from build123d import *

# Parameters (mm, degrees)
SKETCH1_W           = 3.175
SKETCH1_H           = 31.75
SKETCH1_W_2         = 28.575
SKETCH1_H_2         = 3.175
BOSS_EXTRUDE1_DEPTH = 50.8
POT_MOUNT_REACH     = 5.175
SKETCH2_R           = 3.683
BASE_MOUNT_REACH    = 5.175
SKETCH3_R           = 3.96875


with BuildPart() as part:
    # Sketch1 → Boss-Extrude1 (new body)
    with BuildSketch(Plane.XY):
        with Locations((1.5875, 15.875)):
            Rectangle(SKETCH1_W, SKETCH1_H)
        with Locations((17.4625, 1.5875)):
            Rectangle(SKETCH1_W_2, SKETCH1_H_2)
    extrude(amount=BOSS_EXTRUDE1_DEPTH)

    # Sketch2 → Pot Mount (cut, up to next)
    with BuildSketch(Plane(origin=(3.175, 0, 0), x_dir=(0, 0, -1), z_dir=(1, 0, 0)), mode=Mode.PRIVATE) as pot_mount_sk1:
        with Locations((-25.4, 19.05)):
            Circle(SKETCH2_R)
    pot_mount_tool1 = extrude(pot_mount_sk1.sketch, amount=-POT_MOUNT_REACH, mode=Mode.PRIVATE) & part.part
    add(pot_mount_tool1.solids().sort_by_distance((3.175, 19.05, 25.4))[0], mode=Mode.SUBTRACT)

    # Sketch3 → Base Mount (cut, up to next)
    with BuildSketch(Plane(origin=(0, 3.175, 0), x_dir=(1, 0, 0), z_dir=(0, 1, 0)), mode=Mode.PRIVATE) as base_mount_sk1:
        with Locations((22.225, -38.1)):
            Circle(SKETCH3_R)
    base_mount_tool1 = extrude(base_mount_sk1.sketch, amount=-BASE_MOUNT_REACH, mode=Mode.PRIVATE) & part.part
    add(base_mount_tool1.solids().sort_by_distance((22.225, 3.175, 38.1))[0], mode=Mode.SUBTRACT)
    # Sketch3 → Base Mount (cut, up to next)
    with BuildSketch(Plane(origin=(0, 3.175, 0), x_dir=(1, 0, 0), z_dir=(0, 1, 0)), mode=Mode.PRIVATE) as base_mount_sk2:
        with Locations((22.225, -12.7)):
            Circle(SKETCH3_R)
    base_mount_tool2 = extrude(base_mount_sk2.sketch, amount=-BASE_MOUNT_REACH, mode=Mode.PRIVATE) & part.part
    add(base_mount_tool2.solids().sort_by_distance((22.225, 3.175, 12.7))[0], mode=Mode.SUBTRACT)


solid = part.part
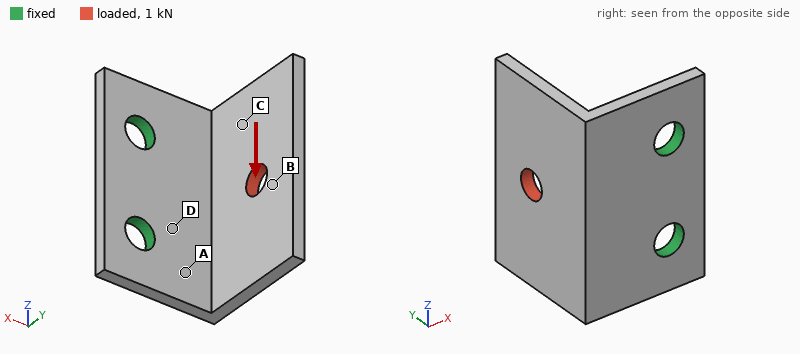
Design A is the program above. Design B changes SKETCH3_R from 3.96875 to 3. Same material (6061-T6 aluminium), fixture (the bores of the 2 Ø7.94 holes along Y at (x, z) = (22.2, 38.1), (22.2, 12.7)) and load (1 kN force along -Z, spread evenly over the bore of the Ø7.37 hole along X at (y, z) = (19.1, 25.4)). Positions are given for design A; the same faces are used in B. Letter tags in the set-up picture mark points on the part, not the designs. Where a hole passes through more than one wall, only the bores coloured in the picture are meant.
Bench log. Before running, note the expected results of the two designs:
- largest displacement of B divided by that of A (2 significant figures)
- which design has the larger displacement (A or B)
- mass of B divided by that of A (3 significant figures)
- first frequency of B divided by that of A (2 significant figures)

1.1
B
1.01
0.96
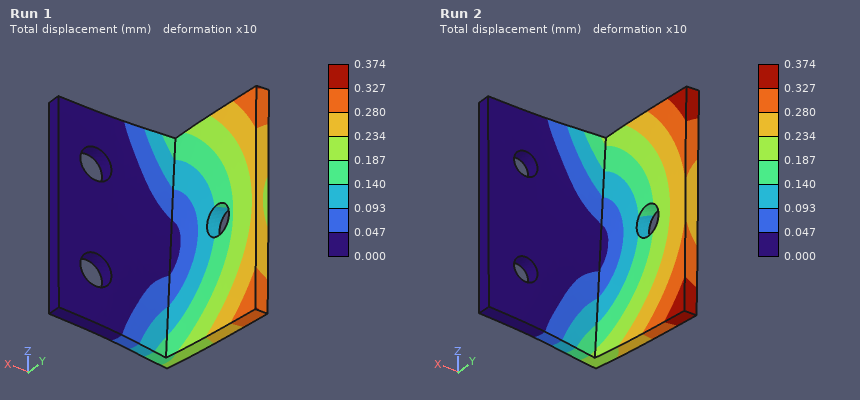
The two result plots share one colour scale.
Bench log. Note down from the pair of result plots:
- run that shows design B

Run 2
